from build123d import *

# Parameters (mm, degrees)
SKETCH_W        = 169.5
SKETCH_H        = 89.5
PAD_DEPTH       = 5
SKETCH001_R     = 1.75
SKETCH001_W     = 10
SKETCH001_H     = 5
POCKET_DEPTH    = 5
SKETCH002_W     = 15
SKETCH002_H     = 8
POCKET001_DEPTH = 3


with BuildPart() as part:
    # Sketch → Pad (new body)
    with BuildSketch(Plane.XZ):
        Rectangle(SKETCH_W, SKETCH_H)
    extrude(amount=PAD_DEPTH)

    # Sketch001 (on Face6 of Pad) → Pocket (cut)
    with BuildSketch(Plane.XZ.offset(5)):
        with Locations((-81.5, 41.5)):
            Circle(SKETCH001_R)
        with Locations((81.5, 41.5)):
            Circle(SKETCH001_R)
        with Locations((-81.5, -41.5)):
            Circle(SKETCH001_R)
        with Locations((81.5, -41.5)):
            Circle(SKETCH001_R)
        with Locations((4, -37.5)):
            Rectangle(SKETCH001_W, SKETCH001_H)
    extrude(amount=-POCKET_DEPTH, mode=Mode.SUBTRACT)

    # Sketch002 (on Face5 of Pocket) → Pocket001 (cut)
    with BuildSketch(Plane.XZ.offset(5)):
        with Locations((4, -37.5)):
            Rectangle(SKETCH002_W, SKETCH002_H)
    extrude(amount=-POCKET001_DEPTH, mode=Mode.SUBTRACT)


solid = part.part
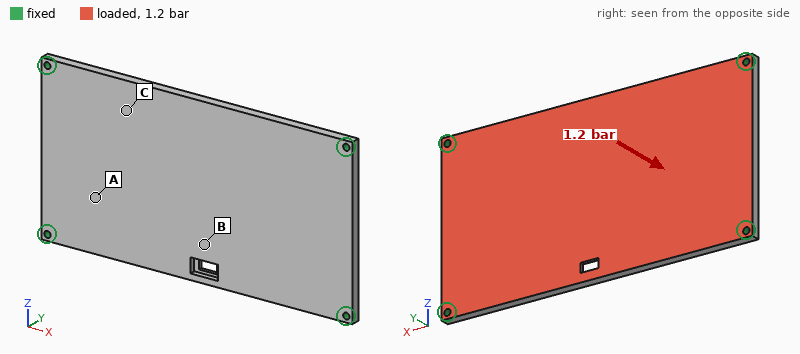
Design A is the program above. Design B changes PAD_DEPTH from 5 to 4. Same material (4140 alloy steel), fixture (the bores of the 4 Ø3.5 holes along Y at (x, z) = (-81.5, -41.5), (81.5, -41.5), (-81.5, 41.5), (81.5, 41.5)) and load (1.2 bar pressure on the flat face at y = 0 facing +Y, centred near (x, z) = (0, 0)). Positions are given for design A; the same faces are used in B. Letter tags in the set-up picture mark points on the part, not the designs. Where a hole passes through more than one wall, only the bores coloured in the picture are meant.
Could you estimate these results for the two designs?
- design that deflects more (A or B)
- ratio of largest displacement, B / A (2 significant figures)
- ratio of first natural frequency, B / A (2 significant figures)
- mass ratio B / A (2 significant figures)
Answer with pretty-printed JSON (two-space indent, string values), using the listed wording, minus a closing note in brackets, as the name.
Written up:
{
  "design that deflects more": "B",
  "ratio of largest displacement, B / A": "1.9",
  "ratio of first natural frequency, B / A": "0.81",
  "mass ratio B / A": "0.80"
}
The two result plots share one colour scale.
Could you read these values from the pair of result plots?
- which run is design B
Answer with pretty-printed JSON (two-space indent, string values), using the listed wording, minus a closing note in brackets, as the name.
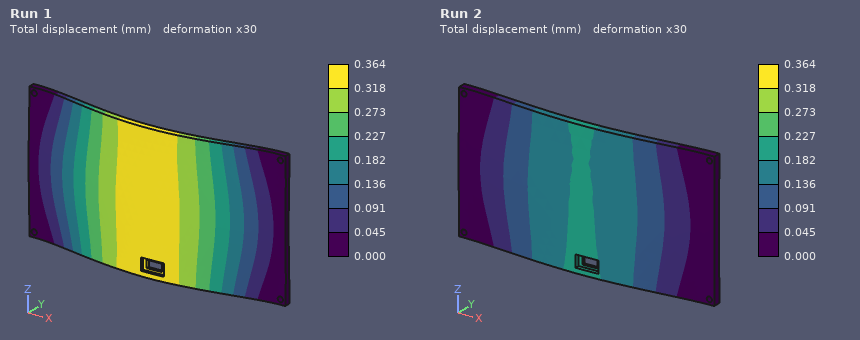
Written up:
{
  "which run is design B": "Run 1"
}
